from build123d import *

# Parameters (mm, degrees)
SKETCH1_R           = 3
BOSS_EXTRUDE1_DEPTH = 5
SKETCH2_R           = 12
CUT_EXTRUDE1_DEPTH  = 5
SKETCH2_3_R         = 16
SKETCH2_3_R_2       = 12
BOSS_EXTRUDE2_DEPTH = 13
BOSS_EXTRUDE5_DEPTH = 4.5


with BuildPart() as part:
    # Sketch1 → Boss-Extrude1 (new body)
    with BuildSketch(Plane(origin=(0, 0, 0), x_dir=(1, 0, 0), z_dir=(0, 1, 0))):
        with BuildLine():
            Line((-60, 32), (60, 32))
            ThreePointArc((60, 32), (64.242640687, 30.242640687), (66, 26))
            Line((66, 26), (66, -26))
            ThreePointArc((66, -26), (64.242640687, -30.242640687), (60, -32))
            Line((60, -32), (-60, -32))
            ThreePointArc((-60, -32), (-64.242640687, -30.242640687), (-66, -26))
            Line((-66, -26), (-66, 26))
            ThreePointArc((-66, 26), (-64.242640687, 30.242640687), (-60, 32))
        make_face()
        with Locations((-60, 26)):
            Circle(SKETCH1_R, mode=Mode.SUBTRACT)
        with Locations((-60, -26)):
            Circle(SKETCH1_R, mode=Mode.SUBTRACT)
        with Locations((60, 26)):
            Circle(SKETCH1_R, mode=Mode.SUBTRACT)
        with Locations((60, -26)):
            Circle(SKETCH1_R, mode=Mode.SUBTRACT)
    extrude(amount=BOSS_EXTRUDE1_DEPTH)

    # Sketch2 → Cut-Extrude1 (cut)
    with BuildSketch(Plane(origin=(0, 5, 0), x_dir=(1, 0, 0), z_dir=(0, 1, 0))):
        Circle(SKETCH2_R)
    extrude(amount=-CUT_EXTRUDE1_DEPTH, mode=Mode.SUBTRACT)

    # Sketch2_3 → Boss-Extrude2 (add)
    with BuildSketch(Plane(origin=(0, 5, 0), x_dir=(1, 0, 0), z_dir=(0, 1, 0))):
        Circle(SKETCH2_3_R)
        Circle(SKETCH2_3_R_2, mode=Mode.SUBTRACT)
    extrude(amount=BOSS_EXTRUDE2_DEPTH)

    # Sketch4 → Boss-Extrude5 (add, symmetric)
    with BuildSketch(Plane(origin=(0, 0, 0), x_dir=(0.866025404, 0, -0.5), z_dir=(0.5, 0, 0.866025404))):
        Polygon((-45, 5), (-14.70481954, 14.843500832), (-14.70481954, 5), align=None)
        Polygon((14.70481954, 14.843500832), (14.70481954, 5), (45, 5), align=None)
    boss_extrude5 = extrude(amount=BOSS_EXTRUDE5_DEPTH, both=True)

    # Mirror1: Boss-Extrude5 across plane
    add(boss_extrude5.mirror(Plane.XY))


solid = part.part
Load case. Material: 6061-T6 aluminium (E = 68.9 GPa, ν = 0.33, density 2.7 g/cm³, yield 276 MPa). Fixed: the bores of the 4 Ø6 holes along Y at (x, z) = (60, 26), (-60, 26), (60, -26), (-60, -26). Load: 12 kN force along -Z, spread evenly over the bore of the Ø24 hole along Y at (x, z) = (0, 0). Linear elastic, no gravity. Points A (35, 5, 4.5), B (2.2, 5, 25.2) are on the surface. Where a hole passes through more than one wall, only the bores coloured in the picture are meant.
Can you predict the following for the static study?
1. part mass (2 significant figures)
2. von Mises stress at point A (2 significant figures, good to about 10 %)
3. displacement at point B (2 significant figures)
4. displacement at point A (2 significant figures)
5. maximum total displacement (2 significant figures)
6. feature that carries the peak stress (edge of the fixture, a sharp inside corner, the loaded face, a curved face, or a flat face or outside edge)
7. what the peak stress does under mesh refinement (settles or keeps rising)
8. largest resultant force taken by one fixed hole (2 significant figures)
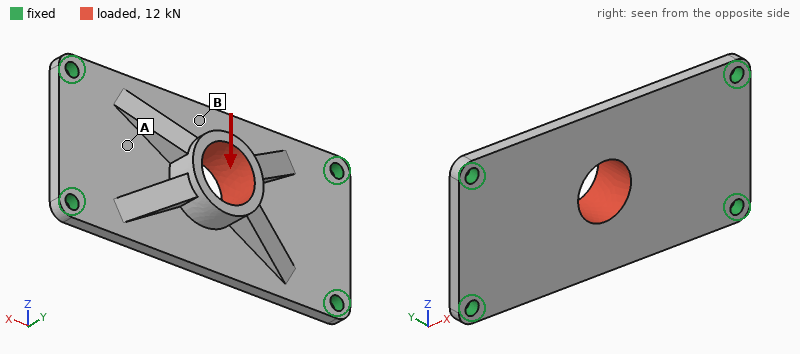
130 g
76 MPa
0.19 mm
0.040 mm
0.24 mm
edge of the fixture
keeps rising
4.7 kN
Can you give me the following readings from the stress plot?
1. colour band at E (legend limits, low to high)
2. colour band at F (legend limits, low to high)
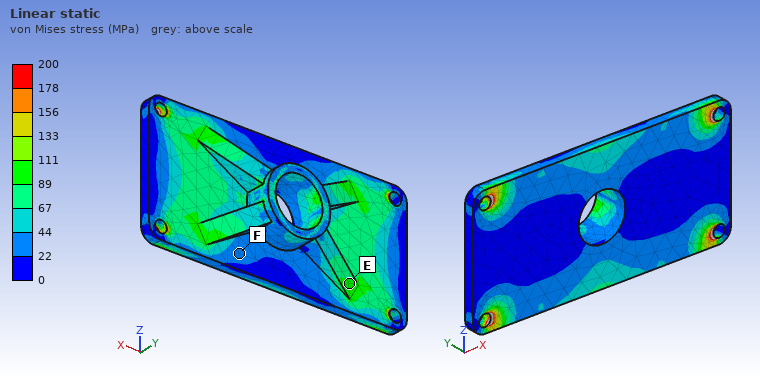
89 to 111 MPa
22 to 44 MPa
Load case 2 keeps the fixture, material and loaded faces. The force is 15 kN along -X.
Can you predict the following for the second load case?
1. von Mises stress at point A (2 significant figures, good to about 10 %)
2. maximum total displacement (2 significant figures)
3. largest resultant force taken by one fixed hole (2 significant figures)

40 MPa
65 µm
3.9 kN
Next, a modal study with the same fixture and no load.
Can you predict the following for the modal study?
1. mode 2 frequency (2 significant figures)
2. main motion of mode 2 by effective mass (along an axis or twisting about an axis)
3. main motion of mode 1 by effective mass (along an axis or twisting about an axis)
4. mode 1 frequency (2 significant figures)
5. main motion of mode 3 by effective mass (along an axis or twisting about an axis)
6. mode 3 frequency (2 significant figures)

3300 Hz
twisting about X
along Y
2100 Hz
twisting about Z
5200 Hz
